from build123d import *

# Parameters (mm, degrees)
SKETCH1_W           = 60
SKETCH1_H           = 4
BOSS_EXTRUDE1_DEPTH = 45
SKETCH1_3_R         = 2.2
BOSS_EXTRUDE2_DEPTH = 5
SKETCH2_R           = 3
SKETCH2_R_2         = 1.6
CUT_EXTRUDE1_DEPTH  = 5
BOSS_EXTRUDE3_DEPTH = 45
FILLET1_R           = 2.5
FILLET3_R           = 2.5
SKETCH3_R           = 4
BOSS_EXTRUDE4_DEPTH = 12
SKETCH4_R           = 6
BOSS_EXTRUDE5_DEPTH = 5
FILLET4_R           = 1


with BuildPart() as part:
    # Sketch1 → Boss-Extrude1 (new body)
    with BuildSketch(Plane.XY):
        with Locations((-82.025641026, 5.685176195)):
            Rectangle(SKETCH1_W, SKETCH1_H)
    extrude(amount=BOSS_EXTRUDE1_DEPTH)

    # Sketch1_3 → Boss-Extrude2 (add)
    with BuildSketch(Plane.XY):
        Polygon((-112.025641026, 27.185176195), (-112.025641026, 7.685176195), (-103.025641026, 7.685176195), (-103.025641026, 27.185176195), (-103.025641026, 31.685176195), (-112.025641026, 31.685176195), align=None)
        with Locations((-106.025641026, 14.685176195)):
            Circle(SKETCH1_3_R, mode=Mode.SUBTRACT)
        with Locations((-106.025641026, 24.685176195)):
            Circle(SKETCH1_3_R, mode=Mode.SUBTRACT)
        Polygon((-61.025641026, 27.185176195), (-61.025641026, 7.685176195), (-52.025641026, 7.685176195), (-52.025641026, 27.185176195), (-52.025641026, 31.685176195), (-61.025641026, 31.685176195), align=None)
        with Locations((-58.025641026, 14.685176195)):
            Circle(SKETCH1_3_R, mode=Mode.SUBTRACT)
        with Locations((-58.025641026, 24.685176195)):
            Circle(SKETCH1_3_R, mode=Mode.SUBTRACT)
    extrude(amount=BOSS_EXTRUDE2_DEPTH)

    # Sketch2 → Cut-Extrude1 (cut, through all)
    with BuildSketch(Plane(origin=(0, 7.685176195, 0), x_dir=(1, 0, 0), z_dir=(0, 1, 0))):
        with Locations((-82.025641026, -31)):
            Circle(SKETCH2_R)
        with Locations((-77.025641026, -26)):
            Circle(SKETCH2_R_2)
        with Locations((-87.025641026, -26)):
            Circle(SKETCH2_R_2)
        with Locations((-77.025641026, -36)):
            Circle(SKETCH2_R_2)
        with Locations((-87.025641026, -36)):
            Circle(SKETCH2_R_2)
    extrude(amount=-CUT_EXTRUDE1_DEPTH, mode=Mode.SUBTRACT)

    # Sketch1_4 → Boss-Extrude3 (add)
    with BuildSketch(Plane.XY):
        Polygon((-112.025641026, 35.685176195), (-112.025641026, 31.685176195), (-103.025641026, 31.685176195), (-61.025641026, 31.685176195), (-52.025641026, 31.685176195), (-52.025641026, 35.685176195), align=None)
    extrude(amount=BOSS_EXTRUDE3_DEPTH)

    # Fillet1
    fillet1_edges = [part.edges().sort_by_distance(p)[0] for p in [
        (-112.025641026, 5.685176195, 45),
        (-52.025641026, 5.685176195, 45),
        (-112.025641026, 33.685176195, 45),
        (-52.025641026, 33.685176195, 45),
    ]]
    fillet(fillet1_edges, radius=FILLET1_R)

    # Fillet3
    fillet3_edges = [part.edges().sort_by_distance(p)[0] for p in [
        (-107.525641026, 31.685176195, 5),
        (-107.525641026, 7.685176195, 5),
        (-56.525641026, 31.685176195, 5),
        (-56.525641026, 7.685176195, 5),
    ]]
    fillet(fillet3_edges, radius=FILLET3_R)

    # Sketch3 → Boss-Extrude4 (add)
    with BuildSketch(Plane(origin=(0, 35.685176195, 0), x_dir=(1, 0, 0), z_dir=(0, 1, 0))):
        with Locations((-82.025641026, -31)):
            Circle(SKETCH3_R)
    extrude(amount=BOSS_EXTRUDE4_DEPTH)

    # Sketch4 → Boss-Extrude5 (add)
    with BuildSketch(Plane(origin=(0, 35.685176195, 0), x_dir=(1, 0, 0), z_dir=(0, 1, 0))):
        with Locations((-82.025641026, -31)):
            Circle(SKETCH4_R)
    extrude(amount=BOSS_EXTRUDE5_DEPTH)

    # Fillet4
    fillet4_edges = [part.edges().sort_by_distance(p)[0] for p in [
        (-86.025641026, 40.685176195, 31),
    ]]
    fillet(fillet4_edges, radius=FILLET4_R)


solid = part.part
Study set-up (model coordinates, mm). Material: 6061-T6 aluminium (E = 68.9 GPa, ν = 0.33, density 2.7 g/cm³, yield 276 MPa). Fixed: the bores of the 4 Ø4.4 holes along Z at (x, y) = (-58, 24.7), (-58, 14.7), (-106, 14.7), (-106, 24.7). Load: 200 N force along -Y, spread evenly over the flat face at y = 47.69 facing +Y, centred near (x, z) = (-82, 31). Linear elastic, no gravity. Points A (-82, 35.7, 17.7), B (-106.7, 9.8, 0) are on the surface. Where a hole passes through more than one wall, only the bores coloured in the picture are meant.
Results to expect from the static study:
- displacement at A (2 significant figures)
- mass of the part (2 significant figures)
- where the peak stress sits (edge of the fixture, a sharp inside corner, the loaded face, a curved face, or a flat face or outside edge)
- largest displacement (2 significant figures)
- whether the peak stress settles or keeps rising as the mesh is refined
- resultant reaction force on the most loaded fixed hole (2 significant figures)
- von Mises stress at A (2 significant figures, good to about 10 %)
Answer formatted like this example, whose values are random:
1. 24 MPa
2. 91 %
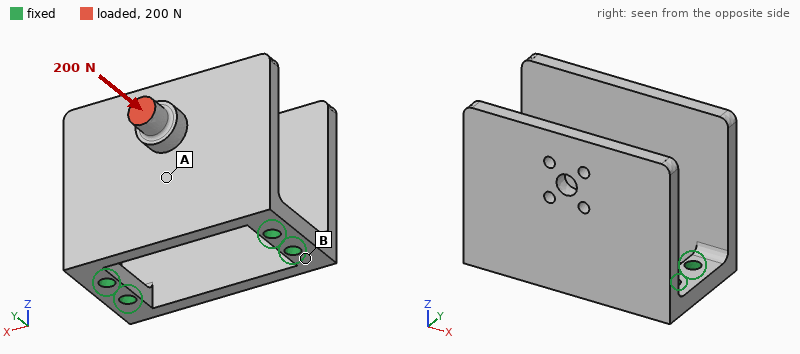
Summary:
1. 0.098 mm
2. 65 g
3. a sharp inside corner
4. 0.30 mm
5. keeps rising
6. 120 N
7. 16 MPa
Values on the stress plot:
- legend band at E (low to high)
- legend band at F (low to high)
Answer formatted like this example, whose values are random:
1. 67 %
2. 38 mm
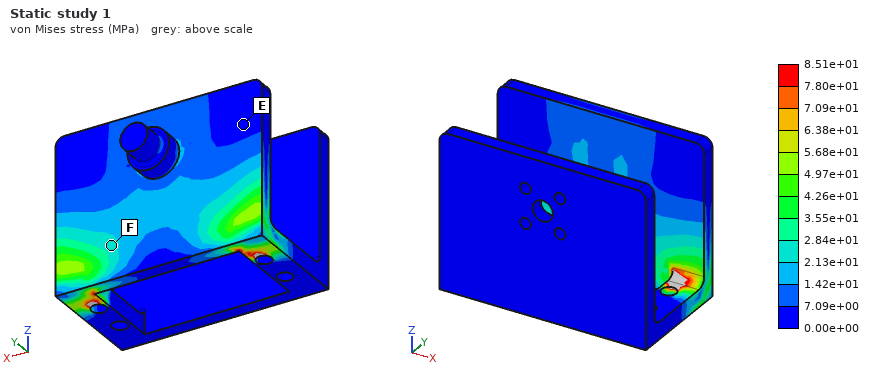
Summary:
1. 0.00e+00 to 7.09e+00 MPa
2. 2.13e+01 to 2.84e+01 MPa
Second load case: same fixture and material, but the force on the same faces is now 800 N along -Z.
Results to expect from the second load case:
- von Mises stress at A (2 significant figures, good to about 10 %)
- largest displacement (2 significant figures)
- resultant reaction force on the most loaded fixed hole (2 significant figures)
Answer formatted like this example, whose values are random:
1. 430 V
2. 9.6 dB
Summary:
1. 68 MPa
2. 0.83 mm
3. 490 N
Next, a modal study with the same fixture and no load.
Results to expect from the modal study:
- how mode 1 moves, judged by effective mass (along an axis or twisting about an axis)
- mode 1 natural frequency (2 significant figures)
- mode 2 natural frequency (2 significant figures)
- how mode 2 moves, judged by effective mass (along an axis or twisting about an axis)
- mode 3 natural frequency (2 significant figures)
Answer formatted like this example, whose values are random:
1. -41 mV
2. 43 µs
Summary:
1. along Y
2. 1100 Hz
3. 1200 Hz
4. along Y
5. 3100 Hz
